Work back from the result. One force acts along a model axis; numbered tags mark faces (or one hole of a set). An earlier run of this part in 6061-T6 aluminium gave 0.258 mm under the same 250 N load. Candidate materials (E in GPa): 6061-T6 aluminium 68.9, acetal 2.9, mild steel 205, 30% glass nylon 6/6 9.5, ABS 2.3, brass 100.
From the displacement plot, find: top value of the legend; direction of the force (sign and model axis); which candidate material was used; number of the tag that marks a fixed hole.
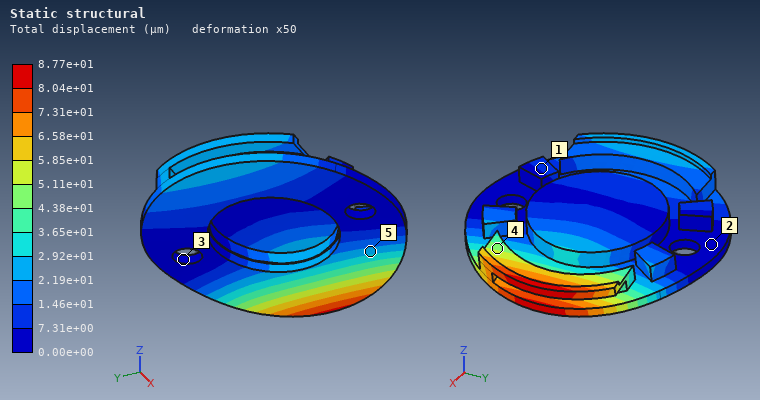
8.77e+01 µm
-Z
mild steel
3
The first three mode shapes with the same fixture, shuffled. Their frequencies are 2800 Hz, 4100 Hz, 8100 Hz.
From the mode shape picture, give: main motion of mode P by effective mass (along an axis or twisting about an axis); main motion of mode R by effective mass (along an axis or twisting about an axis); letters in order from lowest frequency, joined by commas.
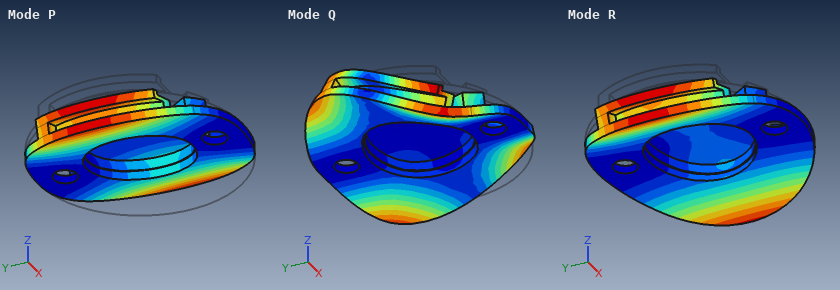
twisting about Y
along Z
P, R, Q
